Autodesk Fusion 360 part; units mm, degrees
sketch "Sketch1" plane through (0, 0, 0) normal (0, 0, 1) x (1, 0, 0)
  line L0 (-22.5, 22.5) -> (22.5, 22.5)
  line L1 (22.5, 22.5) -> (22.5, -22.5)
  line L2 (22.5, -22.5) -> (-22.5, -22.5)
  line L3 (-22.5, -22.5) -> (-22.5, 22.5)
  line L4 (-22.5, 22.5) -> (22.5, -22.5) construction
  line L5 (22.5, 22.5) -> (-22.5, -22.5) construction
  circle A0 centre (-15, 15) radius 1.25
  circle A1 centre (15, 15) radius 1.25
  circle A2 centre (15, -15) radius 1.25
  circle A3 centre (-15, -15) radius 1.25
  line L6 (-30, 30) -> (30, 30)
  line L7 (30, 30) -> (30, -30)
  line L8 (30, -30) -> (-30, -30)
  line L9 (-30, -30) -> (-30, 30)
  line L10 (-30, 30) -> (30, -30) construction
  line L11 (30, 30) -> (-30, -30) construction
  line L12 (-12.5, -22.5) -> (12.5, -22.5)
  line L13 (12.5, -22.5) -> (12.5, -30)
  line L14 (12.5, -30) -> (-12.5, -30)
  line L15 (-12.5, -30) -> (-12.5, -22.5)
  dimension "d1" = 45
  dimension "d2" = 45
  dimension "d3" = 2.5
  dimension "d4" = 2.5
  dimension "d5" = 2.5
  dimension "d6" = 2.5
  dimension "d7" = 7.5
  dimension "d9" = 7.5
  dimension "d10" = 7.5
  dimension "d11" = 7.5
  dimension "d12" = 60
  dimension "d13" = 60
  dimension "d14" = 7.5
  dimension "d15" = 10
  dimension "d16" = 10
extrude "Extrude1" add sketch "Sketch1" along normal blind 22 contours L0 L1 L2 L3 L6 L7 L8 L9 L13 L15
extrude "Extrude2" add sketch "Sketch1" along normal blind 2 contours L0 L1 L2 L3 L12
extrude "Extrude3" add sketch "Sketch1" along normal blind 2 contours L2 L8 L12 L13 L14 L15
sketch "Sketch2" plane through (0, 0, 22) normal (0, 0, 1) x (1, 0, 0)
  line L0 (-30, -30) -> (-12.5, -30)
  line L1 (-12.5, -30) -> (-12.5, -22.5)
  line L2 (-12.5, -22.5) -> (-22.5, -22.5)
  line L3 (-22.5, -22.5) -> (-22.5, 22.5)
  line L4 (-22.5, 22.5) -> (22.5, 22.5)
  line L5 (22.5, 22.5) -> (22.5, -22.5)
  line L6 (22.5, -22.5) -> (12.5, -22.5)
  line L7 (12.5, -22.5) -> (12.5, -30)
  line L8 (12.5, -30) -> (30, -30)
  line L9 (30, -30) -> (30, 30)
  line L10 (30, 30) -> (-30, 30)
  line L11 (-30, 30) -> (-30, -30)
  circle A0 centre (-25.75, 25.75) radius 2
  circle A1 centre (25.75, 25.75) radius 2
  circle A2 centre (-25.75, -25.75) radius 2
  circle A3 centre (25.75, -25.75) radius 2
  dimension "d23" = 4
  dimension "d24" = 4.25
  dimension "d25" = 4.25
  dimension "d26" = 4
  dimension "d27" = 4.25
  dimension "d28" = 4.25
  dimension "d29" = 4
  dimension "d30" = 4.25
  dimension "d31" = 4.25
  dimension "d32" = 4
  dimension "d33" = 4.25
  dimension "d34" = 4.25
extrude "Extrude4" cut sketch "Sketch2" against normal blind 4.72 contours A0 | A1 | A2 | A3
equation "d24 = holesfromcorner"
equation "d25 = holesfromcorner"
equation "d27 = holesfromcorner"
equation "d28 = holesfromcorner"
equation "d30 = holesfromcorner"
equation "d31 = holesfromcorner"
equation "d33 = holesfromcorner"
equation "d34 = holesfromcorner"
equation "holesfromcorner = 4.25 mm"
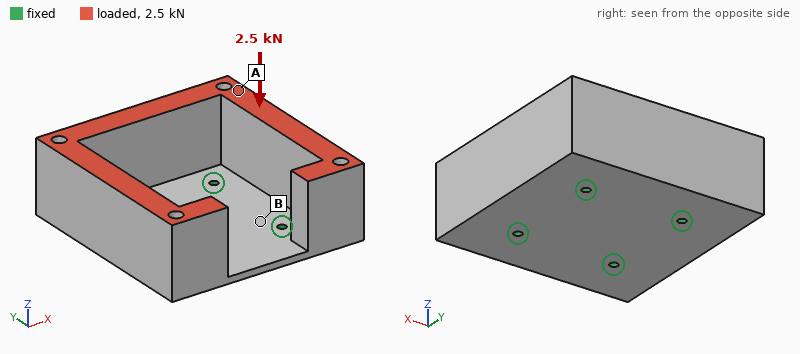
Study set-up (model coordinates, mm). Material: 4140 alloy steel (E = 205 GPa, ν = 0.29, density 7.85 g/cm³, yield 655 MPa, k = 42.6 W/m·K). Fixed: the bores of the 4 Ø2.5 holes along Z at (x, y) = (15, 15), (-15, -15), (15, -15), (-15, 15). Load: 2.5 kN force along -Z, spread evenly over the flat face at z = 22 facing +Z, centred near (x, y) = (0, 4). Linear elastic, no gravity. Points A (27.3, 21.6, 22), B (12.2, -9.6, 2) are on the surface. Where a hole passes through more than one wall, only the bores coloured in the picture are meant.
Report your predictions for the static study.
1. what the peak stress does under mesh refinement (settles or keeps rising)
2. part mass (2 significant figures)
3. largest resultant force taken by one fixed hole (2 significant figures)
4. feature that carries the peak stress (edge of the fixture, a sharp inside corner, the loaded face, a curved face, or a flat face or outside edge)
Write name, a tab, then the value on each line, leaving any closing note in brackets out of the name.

what the peak stress does under mesh refinement	keeps rising
part mass	270 g
largest resultant force taken by one fixed hole	790 N
feature that carries the peak stress	edge of the fixture
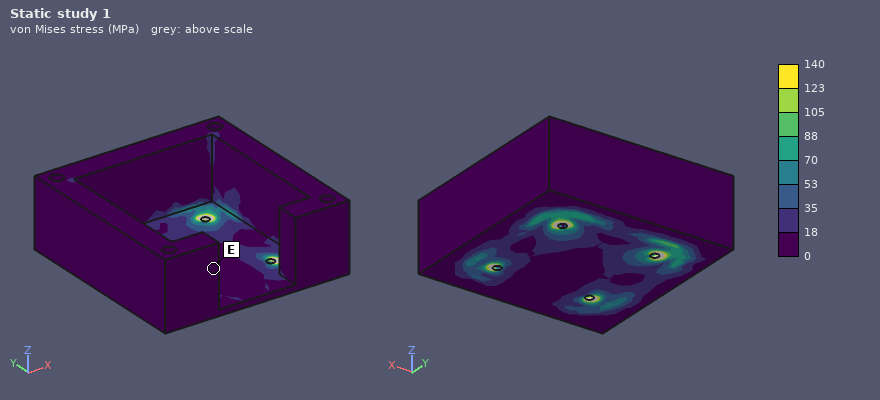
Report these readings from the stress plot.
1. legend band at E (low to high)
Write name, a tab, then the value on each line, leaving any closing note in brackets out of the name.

legend band at E	0 to 18 MPa
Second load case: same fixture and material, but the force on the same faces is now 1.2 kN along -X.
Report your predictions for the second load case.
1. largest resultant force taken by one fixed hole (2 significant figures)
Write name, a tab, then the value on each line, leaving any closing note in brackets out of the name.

largest resultant force taken by one fixed hole	800 N
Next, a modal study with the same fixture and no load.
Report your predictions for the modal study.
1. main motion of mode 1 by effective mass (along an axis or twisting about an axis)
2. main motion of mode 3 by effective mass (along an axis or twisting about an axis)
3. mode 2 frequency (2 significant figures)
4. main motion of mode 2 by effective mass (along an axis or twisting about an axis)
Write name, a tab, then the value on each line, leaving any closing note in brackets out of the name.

main motion of mode 1 by effective mass	along X
main motion of mode 3 by effective mass	along Z
mode 2 frequency	2900 Hz
main motion of mode 2 by effective mass	along Y
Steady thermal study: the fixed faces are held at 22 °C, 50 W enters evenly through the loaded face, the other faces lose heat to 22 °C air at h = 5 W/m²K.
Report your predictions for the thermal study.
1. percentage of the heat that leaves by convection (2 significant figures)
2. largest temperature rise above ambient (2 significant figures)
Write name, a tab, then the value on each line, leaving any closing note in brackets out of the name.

percentage of the heat that leaves by convection	7.7 %
largest temperature rise above ambient	75 K
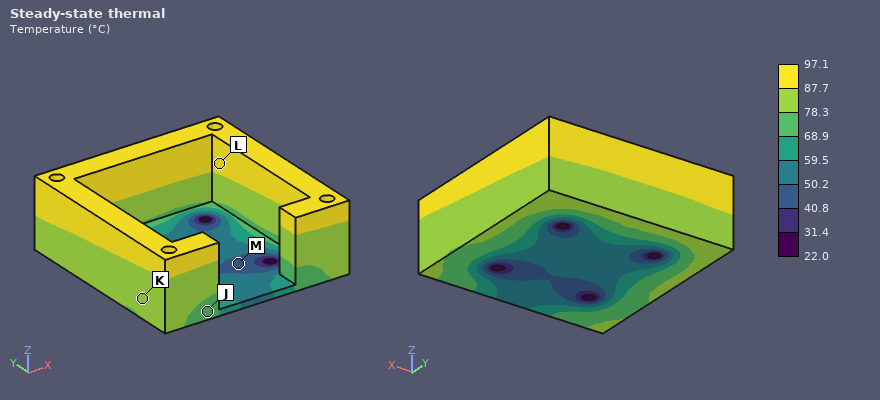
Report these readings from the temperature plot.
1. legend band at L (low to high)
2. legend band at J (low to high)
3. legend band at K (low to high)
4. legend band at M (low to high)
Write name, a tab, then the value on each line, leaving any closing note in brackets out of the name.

legend band at L	87.7 to 97.1 °C
legend band at J	68.9 to 78.3 °C
legend band at K	78.3 to 87.7 °C
legend band at M	40.8 to 50.2 °C
